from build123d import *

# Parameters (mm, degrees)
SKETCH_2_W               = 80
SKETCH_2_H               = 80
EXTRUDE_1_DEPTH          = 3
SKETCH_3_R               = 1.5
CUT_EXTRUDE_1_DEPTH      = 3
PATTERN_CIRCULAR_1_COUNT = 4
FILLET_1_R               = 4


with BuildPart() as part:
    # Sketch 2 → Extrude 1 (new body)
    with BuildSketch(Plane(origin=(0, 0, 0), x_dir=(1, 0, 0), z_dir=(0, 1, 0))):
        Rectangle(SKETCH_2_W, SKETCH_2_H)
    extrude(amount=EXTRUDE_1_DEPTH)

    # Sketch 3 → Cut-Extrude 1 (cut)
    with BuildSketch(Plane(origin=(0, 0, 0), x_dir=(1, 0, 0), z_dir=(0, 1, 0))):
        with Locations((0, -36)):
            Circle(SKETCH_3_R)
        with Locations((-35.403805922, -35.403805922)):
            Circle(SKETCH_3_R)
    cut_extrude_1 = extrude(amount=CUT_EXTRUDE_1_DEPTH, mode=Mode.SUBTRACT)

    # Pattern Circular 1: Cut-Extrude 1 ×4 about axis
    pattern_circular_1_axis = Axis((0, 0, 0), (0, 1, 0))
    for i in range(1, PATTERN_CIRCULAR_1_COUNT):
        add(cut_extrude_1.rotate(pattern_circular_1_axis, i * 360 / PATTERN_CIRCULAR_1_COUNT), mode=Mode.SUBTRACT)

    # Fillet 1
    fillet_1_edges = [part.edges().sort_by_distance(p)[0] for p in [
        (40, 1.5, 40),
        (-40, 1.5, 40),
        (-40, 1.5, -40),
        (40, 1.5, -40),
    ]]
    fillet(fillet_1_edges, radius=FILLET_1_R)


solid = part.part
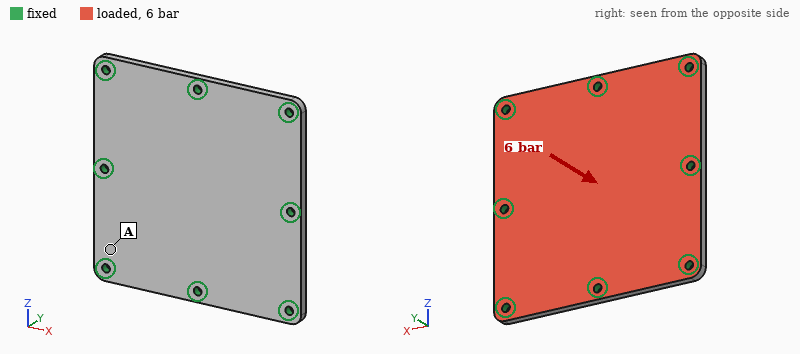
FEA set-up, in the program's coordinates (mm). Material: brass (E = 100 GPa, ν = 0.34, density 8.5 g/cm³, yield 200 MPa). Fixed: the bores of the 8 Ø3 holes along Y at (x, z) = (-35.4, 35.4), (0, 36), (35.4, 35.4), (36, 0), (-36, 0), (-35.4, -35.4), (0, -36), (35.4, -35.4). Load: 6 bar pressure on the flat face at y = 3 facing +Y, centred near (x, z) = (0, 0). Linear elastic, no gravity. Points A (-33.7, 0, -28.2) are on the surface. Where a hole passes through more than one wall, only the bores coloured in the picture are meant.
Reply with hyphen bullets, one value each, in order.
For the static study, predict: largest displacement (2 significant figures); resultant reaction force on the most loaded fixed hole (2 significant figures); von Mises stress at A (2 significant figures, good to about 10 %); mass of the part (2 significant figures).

- 0.12 mm
- 690 N
- 25 MPa
- 160 g
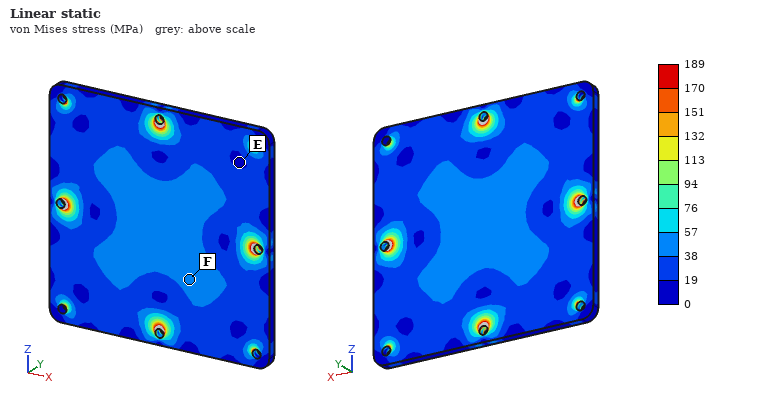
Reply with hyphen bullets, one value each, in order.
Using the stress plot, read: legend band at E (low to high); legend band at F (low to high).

- 0 to 19 MPa
- 38 to 57 MPa
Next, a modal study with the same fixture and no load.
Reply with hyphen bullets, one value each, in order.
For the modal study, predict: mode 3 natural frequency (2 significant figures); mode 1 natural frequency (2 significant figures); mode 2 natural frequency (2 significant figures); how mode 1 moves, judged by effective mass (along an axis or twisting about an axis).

- 5200 Hz
- 2900 Hz
- 5200 Hz
- along Y
